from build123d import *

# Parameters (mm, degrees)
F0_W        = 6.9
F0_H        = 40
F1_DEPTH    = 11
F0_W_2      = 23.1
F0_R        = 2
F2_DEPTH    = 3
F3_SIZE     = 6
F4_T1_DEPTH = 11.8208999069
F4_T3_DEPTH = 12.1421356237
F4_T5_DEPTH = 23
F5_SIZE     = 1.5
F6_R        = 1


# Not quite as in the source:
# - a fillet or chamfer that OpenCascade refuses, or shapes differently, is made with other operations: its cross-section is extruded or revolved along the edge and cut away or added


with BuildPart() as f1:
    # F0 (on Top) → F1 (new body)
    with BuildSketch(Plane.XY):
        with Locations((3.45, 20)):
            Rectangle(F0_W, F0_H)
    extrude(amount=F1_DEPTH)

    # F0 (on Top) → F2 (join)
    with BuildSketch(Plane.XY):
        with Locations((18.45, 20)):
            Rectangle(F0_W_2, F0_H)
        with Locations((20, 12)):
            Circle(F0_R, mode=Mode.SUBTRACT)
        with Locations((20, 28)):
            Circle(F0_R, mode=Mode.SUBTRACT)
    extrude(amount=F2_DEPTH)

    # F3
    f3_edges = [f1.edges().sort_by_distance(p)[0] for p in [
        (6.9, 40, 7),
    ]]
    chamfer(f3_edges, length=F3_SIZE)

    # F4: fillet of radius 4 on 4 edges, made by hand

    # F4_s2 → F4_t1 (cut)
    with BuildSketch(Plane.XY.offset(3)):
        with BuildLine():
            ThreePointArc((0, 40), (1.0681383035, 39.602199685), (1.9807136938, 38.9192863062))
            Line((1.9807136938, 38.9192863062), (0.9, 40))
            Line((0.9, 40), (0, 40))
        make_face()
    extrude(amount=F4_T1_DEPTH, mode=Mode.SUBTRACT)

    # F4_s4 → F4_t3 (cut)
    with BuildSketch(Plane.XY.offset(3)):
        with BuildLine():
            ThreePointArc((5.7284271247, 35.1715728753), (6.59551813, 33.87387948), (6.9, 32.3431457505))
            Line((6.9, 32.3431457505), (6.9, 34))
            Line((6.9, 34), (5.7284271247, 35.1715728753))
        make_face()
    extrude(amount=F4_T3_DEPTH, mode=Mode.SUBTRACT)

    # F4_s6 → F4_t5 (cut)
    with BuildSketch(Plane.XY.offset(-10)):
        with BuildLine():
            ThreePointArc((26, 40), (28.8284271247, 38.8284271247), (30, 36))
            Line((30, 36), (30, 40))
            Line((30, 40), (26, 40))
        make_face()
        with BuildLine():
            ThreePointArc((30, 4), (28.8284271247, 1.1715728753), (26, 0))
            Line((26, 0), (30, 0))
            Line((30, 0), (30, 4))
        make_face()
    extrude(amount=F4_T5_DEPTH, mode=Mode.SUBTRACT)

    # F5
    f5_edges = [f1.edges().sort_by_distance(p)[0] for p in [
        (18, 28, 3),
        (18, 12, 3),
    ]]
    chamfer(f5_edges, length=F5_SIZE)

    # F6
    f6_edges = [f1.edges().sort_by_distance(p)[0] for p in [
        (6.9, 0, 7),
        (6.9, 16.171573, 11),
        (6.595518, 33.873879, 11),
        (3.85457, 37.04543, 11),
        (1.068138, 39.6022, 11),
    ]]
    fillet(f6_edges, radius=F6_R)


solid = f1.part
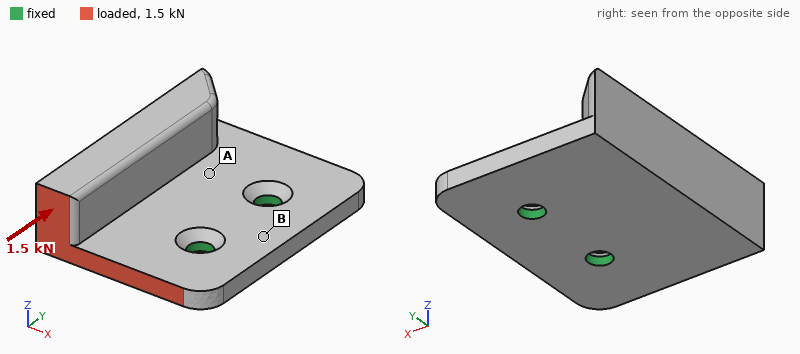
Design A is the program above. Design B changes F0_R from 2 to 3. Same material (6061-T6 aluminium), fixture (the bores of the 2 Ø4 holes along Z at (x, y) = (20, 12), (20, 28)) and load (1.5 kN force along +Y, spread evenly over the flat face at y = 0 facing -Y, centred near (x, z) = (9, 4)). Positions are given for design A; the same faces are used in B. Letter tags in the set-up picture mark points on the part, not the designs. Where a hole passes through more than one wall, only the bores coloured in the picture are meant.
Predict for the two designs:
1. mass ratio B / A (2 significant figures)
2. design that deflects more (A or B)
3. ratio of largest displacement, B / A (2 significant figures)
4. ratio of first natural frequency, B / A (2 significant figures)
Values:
0.98
A
0.84
1.1
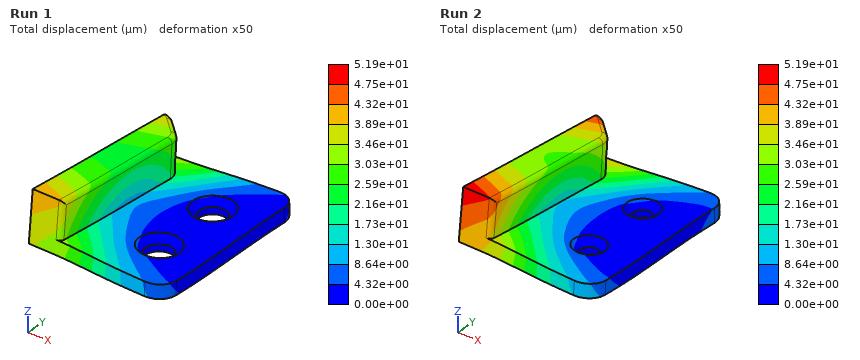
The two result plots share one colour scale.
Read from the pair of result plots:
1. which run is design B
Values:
Run 1
